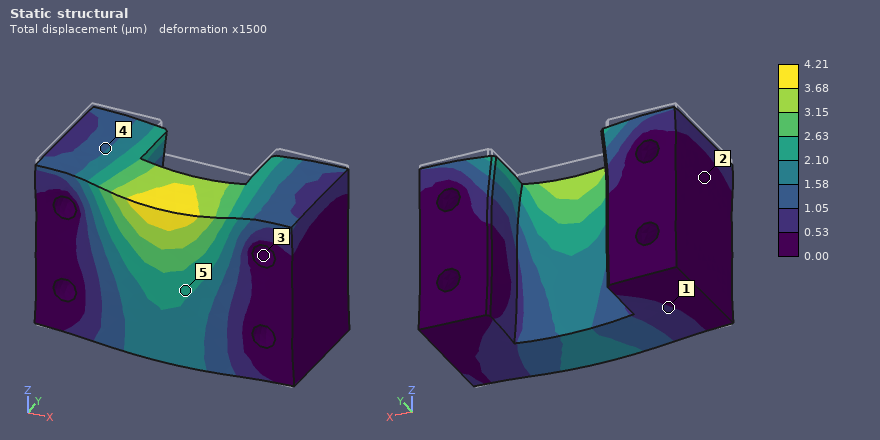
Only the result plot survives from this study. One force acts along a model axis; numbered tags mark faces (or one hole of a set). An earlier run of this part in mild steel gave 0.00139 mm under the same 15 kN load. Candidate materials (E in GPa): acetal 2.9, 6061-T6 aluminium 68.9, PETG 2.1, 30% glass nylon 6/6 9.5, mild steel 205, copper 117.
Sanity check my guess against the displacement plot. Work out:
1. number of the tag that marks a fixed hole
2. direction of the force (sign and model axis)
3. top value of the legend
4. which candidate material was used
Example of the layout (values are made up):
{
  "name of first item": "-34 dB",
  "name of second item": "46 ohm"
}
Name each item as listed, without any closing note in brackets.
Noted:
{
  "number of the tag that marks a fixed hole": "3",
  "direction of the force": "-Z",
  "top value of the legend": "4.21 µm",
  "which candidate material was used": "6061-T6 aluminium"
}
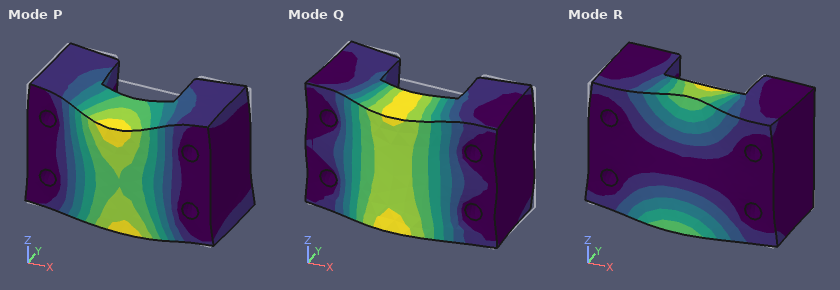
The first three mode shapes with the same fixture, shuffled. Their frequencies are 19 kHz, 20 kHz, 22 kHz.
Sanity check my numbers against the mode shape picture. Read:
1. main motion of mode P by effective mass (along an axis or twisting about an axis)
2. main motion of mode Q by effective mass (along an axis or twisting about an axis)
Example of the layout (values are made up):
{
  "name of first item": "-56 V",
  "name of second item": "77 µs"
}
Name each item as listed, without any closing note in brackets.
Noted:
{
  "main motion of mode P by effective mass": "along Z",
  "main motion of mode Q by effective mass": "along Y"
}
